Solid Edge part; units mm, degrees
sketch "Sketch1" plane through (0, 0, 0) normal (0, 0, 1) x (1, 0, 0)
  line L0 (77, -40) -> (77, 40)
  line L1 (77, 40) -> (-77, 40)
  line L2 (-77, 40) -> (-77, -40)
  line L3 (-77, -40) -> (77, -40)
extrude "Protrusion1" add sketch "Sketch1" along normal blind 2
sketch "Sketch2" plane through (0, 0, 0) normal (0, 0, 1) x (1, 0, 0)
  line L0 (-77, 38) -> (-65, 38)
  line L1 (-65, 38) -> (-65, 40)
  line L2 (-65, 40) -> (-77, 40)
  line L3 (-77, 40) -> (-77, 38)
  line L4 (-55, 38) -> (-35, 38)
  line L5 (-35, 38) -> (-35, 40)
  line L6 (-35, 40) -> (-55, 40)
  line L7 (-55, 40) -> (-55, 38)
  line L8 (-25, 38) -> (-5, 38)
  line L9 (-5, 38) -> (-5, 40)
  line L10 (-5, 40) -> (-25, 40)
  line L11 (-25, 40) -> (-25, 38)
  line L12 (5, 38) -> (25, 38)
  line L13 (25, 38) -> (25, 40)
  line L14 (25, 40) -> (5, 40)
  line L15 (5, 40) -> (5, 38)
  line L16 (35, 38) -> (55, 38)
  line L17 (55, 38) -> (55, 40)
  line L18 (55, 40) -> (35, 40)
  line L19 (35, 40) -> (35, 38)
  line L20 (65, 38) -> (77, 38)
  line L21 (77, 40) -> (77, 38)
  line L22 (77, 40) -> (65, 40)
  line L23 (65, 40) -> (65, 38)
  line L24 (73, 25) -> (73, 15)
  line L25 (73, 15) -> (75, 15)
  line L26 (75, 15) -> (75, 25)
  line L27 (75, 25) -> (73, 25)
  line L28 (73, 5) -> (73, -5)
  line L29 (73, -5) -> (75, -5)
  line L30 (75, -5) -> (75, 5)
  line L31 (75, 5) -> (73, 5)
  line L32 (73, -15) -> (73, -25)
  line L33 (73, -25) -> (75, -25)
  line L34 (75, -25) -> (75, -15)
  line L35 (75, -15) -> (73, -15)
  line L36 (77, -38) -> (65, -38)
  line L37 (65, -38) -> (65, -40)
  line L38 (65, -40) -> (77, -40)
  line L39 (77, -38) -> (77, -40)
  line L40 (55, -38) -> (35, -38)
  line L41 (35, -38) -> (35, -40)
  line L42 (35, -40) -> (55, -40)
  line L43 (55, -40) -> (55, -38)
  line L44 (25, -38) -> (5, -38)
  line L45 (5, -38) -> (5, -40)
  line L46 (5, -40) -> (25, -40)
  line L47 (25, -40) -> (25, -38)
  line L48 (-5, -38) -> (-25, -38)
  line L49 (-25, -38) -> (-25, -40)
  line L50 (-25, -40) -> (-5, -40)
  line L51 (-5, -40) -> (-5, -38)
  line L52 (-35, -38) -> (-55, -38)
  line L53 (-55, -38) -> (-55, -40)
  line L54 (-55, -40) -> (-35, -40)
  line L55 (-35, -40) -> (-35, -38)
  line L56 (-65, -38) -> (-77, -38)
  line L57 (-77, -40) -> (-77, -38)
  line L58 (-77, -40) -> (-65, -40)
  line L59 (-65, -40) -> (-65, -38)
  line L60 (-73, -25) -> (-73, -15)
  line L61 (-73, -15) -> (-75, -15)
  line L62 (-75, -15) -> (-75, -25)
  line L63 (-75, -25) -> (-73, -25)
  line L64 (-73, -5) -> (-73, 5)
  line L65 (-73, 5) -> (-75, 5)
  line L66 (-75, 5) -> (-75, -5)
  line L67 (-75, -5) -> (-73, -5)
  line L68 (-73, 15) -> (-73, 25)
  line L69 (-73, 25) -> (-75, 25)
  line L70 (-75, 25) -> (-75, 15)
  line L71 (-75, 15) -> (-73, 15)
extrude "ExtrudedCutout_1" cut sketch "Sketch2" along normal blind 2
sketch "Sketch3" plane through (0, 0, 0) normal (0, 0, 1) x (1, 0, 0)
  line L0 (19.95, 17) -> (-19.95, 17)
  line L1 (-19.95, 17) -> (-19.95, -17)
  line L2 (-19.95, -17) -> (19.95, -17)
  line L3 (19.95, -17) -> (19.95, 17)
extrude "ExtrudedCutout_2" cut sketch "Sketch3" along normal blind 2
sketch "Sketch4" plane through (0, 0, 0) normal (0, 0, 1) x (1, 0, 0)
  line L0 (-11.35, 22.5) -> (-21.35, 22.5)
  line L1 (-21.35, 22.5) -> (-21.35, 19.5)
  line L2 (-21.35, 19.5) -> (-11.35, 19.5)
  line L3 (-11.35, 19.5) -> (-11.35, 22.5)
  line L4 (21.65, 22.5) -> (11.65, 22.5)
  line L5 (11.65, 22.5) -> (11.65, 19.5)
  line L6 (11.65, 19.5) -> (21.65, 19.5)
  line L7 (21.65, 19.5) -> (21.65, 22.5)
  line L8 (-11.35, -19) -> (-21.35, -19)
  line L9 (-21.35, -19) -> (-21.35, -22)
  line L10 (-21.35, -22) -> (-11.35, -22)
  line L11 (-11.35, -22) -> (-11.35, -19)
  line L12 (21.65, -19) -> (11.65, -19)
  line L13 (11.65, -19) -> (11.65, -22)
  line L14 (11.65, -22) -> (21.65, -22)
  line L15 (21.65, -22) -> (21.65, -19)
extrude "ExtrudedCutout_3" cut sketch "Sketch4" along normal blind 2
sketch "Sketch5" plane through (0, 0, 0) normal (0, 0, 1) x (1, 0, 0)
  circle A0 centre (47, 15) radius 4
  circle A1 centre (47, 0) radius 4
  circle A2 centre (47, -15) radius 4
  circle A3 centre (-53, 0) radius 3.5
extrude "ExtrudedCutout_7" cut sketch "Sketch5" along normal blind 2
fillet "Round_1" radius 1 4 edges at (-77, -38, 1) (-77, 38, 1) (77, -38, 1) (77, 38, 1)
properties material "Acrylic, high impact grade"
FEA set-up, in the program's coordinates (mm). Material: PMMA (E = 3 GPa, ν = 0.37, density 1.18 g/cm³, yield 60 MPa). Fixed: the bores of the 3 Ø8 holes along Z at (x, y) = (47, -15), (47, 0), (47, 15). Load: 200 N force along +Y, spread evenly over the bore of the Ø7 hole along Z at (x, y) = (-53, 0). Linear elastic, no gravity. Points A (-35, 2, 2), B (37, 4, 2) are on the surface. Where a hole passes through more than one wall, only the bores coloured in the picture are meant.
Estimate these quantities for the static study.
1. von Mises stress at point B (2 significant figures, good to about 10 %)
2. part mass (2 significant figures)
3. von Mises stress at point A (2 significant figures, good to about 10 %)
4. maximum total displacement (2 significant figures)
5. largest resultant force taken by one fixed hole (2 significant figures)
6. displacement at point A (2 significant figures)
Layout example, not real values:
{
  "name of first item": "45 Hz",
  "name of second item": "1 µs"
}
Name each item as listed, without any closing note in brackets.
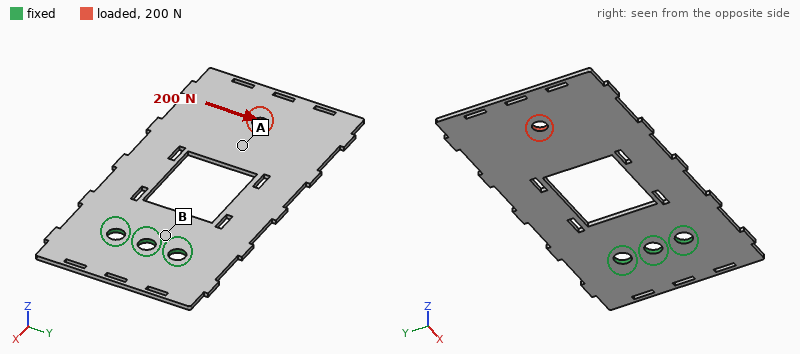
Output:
{
  "von Mises stress at point B": "11 MPa",
  "part mass": "24 g",
  "von Mises stress at point A": "5.4 MPa",
  "maximum total displacement": "1.6 mm",
  "largest resultant force taken by one fixed hole": "520 N",
  "displacement at point A": "1.2 mm"
}
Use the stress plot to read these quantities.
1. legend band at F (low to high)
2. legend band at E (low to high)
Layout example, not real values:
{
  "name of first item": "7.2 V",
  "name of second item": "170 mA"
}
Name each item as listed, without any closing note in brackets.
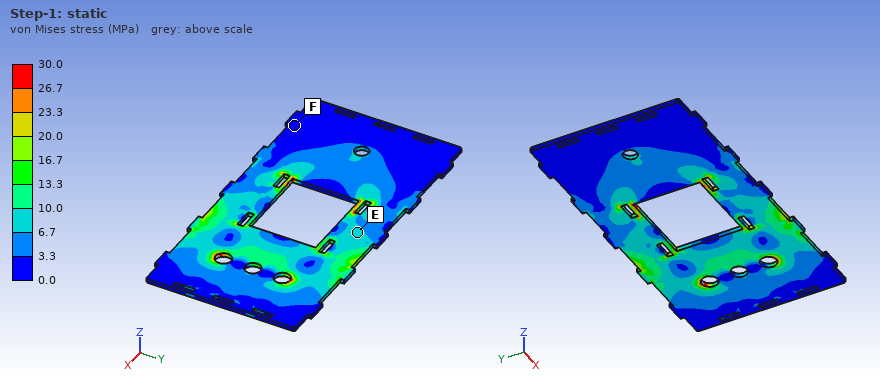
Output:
{
  "legend band at F": "0.0 to 3.3 MPa",
  "legend band at E": "6.7 to 10.0 MPa"
}
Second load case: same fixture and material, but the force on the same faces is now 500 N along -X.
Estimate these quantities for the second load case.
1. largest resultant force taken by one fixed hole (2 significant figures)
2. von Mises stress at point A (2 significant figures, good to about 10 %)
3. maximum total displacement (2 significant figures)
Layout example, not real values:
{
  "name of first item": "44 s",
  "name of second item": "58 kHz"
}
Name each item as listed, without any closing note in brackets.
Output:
{
  "largest resultant force taken by one fixed hole": "230 N",
  "von Mises stress at point A": "3.8 MPa",
  "maximum total displacement": "0.29 mm"
}
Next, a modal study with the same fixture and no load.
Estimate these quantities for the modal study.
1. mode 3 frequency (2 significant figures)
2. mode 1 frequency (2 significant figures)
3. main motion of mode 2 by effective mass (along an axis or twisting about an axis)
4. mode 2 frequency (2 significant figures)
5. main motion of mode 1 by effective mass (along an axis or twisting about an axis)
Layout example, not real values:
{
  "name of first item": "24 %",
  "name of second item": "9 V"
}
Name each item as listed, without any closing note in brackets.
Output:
{
  "mode 3 frequency": "210 Hz",
  "mode 1 frequency": "29 Hz",
  "main motion of mode 2 by effective mass": "twisting about X",
  "mode 2 frequency": "98 Hz",
  "main motion of mode 1 by effective mass": "along Z"
}
